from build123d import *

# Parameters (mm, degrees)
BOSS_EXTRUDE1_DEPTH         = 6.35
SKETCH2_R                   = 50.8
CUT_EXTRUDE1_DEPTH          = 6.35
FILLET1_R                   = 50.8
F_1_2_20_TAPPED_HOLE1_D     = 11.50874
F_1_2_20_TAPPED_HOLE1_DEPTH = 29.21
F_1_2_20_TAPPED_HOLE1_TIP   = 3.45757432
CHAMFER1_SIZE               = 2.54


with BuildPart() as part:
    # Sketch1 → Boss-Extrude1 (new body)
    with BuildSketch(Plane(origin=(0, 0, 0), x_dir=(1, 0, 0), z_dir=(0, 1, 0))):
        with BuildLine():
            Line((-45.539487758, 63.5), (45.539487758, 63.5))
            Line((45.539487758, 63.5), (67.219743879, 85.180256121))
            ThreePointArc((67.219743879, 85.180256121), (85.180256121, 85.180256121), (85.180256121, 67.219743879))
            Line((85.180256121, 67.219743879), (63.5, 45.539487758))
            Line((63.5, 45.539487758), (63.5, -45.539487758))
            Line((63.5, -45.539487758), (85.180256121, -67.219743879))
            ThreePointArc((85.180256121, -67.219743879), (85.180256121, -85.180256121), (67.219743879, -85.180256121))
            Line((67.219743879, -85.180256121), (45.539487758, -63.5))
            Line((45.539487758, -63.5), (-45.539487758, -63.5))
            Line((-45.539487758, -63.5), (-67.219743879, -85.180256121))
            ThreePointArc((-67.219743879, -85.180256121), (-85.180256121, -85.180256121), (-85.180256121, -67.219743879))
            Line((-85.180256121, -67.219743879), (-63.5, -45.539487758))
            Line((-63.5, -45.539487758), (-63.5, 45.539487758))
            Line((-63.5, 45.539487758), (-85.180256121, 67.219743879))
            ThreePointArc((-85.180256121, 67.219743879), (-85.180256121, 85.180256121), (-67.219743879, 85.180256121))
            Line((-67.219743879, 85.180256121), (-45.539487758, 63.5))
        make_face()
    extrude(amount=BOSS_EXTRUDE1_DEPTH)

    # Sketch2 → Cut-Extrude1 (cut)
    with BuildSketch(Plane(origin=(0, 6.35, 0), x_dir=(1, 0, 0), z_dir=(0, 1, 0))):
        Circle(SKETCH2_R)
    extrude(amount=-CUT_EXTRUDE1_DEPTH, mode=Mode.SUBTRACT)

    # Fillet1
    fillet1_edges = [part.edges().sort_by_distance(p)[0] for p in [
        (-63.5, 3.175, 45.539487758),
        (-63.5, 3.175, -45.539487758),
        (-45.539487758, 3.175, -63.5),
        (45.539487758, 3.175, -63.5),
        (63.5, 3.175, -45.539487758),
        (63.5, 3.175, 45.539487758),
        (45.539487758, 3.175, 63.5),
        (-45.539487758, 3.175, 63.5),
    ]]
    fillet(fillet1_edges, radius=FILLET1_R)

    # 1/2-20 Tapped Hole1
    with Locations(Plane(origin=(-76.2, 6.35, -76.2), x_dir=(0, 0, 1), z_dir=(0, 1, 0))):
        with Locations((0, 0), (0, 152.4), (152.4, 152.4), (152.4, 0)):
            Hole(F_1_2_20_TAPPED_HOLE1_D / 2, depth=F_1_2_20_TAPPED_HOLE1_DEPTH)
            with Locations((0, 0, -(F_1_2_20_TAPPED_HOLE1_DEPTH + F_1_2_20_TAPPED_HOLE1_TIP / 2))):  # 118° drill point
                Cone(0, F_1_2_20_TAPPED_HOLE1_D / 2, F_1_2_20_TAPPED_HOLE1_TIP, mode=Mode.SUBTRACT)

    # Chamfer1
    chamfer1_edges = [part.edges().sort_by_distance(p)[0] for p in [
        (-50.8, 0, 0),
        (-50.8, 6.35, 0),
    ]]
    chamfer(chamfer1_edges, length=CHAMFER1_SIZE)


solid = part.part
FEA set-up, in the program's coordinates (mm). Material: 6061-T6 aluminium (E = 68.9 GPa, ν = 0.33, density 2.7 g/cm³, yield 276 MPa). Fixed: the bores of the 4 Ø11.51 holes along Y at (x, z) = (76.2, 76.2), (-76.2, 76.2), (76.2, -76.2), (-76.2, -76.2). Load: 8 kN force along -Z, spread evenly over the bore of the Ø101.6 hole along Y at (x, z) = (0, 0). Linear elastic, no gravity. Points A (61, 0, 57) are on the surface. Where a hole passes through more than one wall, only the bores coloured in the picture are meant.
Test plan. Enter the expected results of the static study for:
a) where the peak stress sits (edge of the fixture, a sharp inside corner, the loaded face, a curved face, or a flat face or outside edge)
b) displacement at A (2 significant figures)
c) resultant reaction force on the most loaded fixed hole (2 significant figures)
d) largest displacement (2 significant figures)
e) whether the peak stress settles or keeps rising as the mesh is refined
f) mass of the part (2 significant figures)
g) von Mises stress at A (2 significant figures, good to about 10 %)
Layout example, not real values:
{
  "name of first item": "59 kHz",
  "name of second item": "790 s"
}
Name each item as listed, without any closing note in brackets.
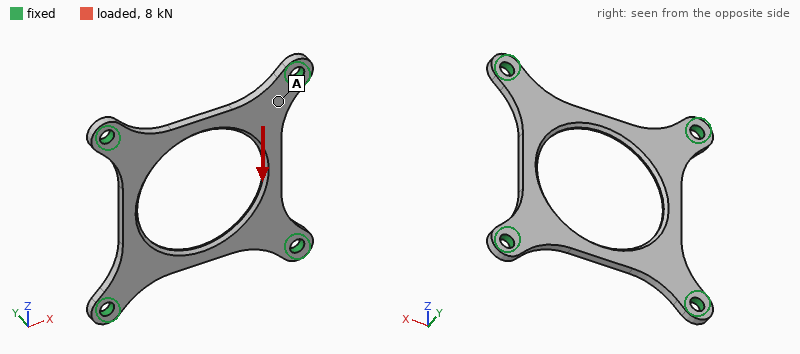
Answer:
{
  "where the peak stress sits": "a sharp inside corner",
  "displacement at A": "13 µm",
  "resultant reaction force on the most loaded fixed hole": "2.4 kN",
  "largest displacement": "74 µm",
  "whether the peak stress settles or keeps rising as the mesh is refined": "keeps rising",
  "mass of the part": "190 g",
  "von Mises stress at A": "13 MPa"
}
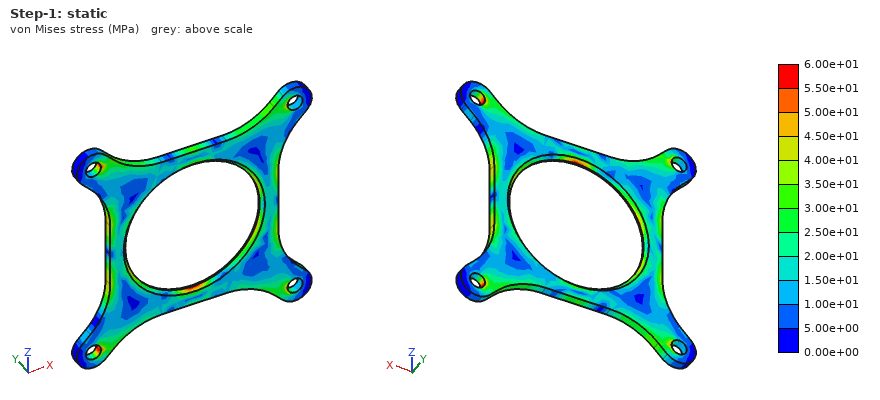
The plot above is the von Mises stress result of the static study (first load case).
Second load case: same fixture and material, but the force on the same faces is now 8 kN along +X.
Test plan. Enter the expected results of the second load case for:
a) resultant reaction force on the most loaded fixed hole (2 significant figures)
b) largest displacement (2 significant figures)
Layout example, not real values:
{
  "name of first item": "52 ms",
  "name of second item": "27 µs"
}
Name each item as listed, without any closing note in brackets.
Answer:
{
  "resultant reaction force on the most loaded fixed hole": "2.4 kN",
  "largest displacement": "75 µm"
}
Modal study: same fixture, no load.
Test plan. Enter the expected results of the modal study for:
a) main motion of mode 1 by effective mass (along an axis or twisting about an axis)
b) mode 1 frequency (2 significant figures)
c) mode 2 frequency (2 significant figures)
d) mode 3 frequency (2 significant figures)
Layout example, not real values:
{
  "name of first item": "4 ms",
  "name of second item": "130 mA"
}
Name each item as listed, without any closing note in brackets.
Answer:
{
  "main motion of mode 1 by effective mass": "along Y",
  "mode 1 frequency": "1200 Hz",
  "mode 2 frequency": "1700 Hz",
  "mode 3 frequency": "1700 Hz"
}
